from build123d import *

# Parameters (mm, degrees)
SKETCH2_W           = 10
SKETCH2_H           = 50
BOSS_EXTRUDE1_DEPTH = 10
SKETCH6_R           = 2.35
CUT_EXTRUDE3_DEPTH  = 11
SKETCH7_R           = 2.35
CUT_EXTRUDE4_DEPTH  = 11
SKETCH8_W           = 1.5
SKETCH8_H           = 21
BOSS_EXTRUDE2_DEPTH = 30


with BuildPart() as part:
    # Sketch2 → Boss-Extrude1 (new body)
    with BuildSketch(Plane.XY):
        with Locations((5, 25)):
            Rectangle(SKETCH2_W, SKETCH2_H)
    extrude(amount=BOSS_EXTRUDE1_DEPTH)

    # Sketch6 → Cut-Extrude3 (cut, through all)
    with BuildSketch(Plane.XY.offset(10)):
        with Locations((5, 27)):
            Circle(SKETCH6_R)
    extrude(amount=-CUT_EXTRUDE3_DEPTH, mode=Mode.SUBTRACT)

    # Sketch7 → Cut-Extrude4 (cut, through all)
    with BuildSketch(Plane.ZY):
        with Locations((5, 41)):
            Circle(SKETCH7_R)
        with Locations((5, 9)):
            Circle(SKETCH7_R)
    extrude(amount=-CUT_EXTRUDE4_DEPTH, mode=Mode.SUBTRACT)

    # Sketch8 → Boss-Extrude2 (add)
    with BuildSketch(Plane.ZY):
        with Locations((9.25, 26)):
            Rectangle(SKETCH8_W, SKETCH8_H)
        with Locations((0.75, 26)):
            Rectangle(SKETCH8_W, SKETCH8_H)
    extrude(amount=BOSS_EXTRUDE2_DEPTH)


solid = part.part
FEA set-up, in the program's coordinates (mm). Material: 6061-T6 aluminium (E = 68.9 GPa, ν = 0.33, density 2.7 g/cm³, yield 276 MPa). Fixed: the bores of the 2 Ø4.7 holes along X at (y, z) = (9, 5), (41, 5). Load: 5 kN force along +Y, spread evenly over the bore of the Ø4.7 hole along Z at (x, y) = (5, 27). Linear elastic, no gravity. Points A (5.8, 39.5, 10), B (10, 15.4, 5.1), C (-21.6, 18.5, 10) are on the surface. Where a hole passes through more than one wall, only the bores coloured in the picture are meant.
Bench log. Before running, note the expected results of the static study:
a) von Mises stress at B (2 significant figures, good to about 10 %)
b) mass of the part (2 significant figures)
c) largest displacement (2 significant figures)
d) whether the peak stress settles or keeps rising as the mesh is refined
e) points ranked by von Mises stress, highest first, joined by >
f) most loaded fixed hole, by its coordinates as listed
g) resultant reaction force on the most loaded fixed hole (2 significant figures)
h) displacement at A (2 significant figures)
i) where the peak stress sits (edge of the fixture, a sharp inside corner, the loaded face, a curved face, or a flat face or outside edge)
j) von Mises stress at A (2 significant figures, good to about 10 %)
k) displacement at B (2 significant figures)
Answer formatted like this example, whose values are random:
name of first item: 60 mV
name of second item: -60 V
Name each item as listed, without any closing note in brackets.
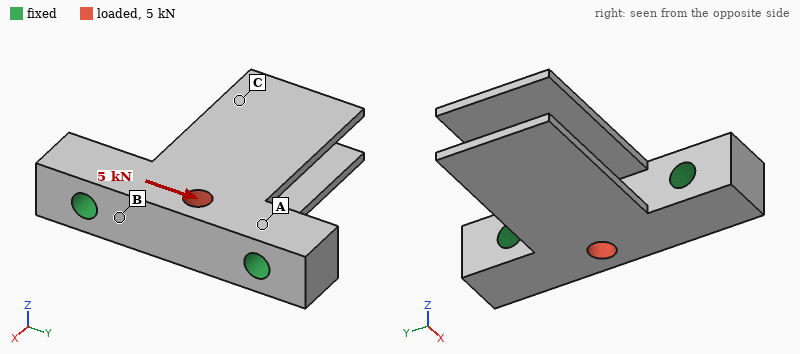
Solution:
von Mises stress at B: 26 MPa
mass of the part: 17 g
largest displacement: 5.8 µm
whether the peak stress settles or keeps rising as the mesh is refined: keeps rising
points ranked by von Mises stress, highest first, joined by >: B > A > C
most loaded fixed hole, by its coordinates as listed: (41, 5)
resultant reaction force on the most loaded fixed hole: 2.8 kN
displacement at A: 1.1 µm
where the peak stress sits: edge of the fixture
von Mises stress at A: 13 MPa
displacement at B: 1.8 µm
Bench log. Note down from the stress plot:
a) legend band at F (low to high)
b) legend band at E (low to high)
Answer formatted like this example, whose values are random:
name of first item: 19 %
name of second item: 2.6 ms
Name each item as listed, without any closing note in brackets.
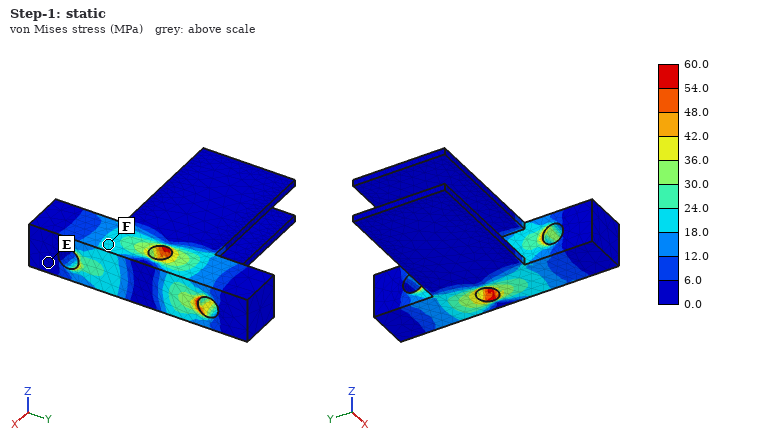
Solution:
legend band at F: 18.0 to 24.0 MPa
legend band at E: 0.0 to 6.0 MPa
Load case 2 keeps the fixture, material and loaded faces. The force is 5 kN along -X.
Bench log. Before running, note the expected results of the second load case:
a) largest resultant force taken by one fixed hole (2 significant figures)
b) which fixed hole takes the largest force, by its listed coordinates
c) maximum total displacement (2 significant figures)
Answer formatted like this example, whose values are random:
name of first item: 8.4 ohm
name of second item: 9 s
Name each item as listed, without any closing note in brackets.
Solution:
largest resultant force taken by one fixed hole: 2.9 kN
which fixed hole takes the largest force, by its listed coordinates: (41, 5)
maximum total displacement: 23 µm
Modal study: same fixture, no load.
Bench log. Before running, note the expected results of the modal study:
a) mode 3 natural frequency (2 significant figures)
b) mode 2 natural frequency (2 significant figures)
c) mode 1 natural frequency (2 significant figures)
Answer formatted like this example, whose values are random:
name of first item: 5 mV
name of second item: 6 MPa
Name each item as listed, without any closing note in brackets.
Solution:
mode 3 natural frequency: 4200 Hz
mode 2 natural frequency: 1300 Hz
mode 1 natural frequency: 1300 Hz
